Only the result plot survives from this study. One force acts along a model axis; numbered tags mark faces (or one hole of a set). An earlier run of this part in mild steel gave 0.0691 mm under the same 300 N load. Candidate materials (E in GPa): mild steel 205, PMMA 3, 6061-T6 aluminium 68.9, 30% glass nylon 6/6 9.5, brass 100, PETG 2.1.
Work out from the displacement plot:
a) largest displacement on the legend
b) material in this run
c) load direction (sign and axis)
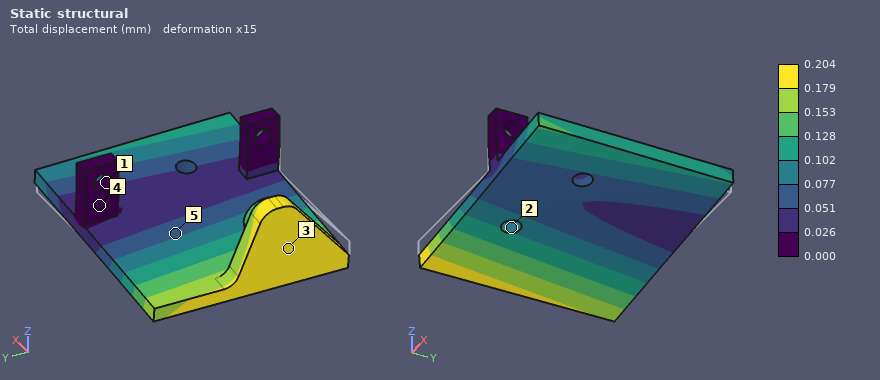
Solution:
0.204 mm
6061-T6 aluminium
+X
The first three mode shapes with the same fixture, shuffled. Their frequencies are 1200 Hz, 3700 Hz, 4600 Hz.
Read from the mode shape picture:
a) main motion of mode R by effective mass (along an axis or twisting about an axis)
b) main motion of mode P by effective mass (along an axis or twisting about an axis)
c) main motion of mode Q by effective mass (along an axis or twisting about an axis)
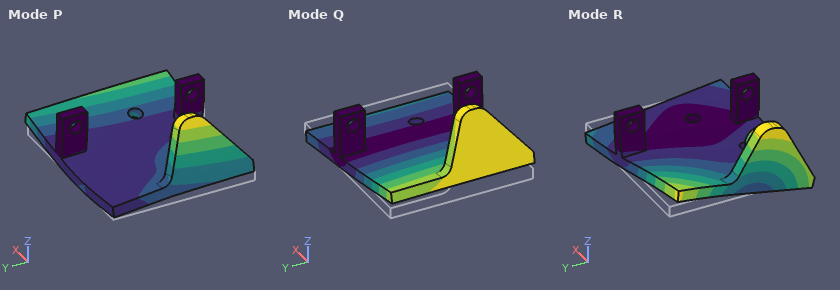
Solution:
along Y
along X
along Z
